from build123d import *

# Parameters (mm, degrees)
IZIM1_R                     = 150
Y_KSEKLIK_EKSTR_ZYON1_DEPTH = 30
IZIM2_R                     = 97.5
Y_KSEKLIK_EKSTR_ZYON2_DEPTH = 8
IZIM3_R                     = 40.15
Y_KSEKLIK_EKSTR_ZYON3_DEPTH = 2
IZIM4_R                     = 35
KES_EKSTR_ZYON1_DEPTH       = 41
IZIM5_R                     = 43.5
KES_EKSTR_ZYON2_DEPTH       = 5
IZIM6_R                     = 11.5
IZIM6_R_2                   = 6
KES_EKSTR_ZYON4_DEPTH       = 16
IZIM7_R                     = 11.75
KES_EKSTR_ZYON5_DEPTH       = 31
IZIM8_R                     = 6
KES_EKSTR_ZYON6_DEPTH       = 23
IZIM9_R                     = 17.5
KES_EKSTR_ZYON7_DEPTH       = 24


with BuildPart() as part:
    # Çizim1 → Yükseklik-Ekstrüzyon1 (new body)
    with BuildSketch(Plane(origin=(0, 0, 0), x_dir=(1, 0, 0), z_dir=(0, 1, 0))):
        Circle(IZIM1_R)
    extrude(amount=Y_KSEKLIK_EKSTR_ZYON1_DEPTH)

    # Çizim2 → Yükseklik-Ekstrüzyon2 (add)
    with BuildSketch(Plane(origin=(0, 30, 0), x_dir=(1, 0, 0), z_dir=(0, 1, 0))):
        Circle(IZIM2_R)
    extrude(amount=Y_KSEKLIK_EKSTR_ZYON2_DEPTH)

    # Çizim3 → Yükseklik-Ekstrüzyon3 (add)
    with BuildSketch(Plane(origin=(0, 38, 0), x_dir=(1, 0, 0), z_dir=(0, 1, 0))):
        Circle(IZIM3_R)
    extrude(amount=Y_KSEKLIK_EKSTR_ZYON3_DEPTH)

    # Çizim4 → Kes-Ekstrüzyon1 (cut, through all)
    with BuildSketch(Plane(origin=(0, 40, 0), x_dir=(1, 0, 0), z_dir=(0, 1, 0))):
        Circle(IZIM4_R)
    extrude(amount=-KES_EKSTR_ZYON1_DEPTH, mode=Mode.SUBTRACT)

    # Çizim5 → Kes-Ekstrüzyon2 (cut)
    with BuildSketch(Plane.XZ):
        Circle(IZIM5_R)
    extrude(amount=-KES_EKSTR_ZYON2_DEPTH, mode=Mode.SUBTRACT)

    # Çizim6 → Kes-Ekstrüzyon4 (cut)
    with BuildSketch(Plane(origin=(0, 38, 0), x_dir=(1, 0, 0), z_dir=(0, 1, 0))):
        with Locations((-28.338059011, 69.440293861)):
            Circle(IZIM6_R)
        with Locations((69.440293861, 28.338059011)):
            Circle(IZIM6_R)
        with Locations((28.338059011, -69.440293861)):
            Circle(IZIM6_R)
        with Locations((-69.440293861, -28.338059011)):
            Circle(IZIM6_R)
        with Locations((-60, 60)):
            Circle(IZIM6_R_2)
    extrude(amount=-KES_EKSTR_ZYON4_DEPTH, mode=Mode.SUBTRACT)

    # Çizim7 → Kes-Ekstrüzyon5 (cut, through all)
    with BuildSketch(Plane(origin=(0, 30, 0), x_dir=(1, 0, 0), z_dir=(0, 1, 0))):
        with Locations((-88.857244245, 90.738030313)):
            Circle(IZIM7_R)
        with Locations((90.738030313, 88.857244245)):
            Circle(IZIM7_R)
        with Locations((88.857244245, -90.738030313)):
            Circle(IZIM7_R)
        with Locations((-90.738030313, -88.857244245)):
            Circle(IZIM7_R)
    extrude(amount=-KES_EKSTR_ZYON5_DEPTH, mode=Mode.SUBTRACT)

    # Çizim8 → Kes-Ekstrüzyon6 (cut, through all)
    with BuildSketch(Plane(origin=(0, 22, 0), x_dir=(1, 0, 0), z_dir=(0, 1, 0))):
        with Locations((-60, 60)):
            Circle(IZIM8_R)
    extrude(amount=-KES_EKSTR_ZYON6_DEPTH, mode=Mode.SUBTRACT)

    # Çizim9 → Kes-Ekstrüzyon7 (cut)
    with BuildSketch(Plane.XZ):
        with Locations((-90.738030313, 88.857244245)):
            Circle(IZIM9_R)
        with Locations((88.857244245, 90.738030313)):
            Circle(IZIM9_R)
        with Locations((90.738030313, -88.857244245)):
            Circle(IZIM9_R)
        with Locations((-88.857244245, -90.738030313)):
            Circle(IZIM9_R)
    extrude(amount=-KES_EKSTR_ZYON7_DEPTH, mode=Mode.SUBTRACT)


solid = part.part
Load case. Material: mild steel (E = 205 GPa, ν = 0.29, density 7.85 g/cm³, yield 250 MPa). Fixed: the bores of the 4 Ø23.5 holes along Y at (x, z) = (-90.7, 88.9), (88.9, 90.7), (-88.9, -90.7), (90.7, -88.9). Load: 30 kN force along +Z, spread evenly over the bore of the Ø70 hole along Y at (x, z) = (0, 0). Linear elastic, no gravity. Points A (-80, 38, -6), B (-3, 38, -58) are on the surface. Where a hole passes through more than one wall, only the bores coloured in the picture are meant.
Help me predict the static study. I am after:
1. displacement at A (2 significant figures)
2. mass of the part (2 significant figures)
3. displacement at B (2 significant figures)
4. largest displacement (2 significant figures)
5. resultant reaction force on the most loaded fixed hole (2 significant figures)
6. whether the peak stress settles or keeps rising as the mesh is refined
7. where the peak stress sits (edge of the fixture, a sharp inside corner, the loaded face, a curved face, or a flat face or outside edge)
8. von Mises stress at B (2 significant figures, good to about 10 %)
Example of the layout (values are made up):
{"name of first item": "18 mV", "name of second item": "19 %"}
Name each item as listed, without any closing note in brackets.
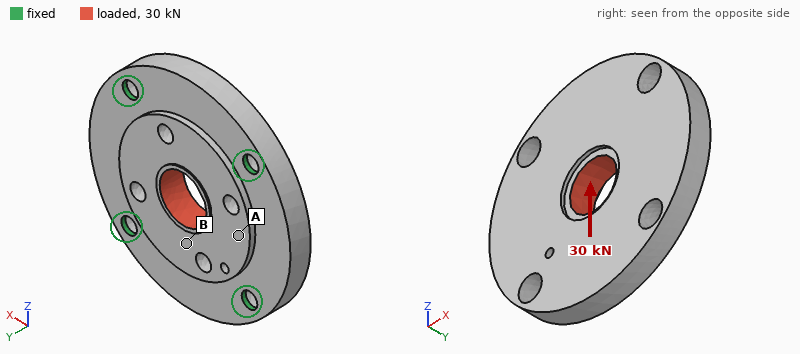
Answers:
{"displacement at A": "2.5 µm", "mass of the part": "16 kg", "displacement at B": "3.5 µm", "largest displacement": "4.2 µm", "resultant reaction force on the most loaded fixed hole": "7.7 kN", "whether the peak stress settles or keeps rising as the mesh is refined": "keeps rising", "where the peak stress sits": "edge of the fixture", "von Mises stress at B": "5.2 MPa"}
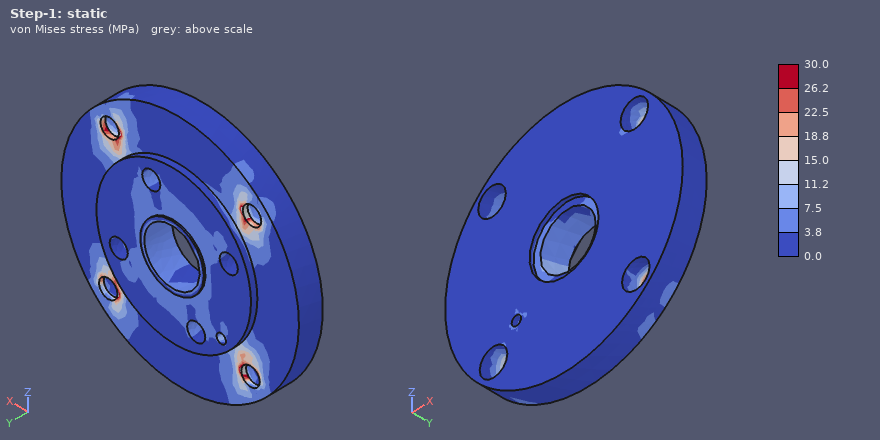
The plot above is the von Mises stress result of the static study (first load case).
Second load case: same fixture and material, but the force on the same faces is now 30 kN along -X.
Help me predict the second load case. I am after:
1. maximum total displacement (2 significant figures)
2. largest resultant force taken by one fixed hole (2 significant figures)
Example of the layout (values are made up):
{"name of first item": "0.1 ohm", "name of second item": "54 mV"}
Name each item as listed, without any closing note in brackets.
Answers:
{"maximum total displacement": "4.2 µm", "largest resultant force taken by one fixed hole": "7.7 kN"}
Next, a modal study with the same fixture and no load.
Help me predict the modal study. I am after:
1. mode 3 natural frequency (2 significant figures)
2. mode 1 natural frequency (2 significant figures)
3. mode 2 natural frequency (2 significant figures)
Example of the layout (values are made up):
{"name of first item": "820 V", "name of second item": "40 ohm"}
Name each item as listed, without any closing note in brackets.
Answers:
{"mode 3 natural frequency": "2700 Hz", "mode 1 natural frequency": "2400 Hz", "mode 2 natural frequency": "2500 Hz"}
